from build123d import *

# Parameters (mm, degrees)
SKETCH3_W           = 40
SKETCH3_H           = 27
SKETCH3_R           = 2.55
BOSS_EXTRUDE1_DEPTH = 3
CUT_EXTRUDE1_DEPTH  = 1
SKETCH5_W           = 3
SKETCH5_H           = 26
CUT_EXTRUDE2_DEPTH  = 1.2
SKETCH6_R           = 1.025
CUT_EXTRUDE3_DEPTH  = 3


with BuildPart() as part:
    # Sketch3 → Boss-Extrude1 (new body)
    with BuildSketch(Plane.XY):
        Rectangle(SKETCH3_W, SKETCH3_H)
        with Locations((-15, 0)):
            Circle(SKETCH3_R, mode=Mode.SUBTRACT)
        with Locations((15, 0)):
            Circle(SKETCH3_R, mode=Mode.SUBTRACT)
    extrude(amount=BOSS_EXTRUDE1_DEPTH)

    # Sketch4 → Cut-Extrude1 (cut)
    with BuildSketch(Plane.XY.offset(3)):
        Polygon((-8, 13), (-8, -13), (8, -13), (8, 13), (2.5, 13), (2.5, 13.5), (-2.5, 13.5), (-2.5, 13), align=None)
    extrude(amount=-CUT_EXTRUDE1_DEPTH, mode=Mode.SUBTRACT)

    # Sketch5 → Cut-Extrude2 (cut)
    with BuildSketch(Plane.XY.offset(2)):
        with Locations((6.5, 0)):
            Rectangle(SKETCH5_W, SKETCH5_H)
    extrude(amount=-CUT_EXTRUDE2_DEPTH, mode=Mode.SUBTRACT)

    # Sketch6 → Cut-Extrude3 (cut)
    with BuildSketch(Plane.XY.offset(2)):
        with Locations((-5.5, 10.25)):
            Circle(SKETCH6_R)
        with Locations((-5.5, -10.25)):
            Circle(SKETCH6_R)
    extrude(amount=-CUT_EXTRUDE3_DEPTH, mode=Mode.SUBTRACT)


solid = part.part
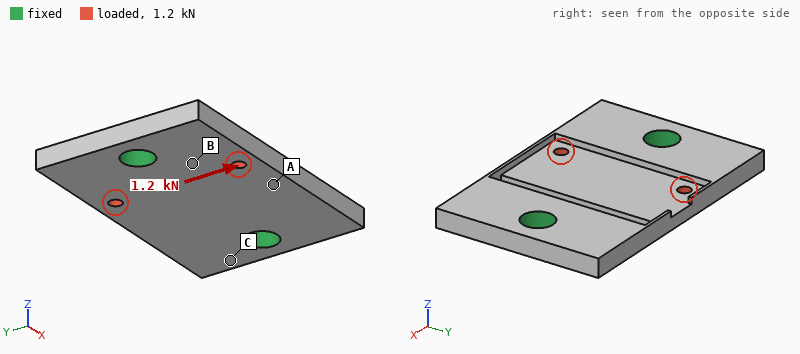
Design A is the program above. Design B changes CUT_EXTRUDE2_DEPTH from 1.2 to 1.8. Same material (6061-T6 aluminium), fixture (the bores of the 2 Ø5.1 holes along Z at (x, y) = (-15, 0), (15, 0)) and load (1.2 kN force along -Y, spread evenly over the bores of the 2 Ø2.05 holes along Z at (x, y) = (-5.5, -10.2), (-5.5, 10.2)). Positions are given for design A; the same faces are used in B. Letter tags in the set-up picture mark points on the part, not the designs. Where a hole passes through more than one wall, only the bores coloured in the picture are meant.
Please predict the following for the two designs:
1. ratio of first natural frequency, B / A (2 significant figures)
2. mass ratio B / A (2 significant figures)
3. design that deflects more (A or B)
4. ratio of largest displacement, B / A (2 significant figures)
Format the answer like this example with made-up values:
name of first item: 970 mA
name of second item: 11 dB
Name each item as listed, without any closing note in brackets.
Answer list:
ratio of first natural frequency, B / A: 1.0
mass ratio B / A: 0.98
design that deflects more: B
ratio of largest displacement, B / A: 1.2
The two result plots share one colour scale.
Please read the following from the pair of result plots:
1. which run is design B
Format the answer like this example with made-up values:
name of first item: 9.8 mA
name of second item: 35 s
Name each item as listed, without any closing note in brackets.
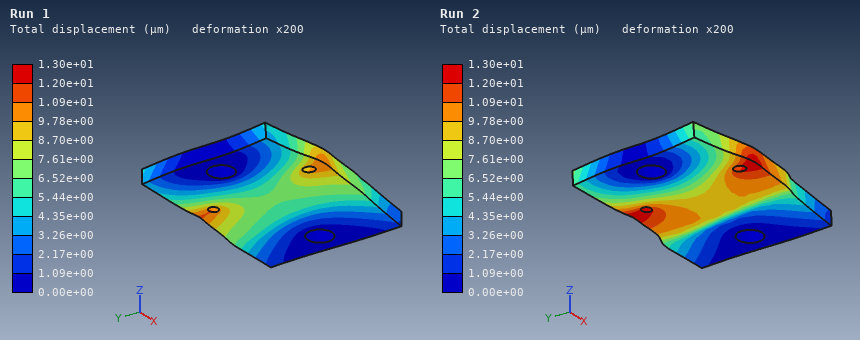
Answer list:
which run is design B: Run 2
